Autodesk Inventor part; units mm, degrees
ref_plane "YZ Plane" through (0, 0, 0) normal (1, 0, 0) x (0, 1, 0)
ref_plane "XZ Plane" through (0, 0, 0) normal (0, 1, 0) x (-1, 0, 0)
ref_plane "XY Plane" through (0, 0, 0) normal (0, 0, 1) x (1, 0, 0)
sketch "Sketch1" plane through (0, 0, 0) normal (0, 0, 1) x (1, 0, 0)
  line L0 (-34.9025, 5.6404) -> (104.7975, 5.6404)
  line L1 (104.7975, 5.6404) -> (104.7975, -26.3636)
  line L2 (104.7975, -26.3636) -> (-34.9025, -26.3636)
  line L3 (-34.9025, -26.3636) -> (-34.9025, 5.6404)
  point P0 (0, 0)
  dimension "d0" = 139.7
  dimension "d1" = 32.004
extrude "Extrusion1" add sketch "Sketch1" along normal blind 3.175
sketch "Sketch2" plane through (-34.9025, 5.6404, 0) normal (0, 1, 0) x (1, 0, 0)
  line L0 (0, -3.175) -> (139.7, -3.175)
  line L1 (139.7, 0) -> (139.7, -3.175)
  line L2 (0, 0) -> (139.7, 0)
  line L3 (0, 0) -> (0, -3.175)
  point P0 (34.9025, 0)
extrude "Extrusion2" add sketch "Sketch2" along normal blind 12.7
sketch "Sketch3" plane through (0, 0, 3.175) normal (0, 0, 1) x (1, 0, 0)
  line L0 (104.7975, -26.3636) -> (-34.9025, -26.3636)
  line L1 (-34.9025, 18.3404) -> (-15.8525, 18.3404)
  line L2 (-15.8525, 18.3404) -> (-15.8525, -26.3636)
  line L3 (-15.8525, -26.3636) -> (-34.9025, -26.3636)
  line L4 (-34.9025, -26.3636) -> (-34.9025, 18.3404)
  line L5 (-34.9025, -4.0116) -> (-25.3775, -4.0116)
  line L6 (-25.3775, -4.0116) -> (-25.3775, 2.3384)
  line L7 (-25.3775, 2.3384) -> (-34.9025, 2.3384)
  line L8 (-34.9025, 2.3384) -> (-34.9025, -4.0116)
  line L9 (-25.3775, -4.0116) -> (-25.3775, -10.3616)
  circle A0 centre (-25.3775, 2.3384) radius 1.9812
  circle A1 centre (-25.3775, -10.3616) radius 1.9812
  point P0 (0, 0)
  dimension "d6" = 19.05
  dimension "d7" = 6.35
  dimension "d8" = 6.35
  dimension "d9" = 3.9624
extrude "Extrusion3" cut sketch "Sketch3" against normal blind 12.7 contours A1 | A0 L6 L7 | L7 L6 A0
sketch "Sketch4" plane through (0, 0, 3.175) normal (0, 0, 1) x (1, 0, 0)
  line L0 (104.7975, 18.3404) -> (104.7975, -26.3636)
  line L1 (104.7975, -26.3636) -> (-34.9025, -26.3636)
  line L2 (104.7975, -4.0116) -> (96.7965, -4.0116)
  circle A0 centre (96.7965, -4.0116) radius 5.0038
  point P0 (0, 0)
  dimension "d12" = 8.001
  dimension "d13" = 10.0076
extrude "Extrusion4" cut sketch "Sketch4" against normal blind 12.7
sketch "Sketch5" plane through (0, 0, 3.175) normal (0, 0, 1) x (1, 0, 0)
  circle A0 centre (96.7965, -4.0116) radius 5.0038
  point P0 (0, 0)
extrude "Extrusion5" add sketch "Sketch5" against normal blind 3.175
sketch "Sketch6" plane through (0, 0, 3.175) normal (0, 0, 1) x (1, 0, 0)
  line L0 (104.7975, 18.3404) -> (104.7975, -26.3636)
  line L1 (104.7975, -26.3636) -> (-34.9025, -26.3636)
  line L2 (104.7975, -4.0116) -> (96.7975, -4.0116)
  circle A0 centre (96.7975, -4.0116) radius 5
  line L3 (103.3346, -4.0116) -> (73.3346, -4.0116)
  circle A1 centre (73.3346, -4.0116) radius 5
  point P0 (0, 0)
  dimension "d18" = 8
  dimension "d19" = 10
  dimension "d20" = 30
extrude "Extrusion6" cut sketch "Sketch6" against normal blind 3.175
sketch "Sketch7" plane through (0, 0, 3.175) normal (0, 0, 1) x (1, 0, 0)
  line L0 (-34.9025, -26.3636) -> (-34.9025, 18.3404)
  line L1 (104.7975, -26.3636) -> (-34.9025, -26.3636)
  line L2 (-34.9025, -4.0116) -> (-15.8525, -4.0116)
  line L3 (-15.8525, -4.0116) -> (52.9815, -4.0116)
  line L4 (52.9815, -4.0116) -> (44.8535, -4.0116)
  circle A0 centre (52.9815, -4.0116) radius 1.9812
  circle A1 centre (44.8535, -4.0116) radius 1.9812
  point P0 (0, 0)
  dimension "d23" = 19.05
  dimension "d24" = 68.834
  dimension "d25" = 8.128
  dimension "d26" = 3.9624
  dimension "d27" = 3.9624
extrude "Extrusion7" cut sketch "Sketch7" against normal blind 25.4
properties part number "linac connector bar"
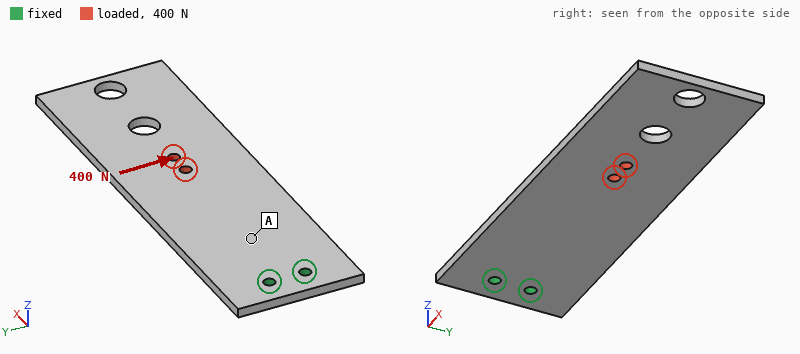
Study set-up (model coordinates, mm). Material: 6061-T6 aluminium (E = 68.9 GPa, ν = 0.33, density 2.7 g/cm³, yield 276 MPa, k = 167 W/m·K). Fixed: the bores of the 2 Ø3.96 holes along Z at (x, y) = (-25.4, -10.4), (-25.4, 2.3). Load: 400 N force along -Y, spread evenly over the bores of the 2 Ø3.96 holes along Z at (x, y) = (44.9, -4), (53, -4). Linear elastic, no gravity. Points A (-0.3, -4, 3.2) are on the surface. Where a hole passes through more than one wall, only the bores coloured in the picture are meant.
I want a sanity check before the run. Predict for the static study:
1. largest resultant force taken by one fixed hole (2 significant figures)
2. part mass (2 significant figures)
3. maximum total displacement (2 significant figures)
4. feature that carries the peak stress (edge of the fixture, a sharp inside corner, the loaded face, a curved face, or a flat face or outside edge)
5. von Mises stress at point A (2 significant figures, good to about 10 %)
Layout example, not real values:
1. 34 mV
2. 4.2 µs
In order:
1. 1.9 kN
2. 52 g
3. 0.18 mm
4. edge of the fixture
5. 9.0 MPa
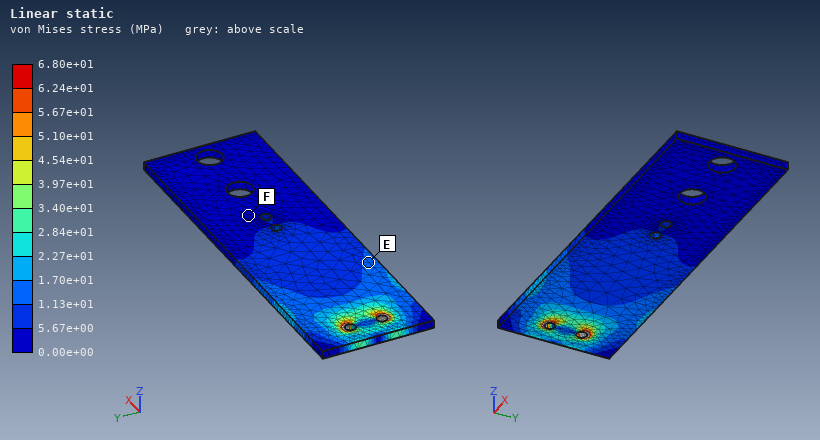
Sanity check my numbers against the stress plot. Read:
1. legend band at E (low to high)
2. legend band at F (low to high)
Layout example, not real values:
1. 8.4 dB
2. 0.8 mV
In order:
1. 1.13e+01 to 1.70e+01 MPa
2. 0.00e+00 to 5.67e+00 MPa
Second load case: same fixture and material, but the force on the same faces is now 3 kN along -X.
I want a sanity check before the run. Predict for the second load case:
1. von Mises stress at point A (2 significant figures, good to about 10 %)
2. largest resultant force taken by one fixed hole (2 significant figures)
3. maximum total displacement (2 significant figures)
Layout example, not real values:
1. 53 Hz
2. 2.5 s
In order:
1. 26 MPa
2. 1.5 kN
3. 33 µm
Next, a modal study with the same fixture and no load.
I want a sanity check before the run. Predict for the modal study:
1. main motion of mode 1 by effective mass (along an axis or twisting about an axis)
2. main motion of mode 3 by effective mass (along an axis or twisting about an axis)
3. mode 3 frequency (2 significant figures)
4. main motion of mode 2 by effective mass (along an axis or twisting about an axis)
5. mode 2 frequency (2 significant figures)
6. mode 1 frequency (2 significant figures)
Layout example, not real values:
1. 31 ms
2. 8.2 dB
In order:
1. along Z
2. along Z
3. 960 Hz
4. twisting about X
5. 860 Hz
6. 160 Hz
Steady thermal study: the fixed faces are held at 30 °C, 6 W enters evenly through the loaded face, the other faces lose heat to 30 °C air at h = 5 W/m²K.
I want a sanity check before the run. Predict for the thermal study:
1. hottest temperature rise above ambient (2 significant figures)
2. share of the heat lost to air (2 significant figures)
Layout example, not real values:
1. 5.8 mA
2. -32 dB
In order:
1. 19 K
2. 13 %
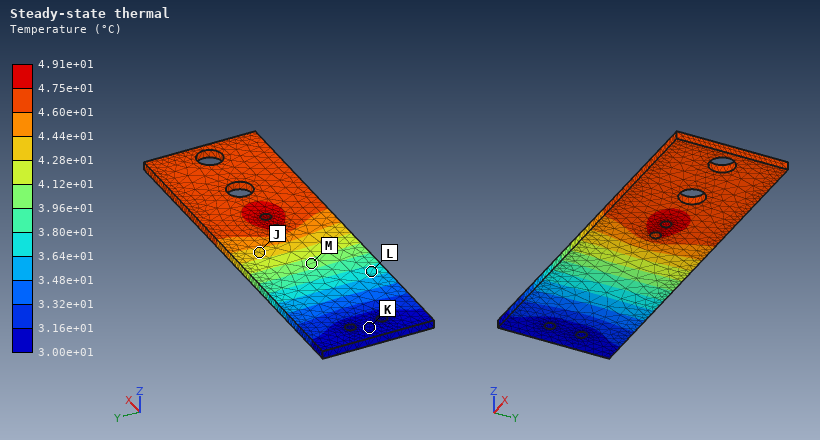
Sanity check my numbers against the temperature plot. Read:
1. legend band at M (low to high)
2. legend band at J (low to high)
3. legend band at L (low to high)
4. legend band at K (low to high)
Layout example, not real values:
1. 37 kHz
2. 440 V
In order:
1. 3.96e+01 to 4.12e+01 °C
2. 4.28e+01 to 4.44e+01 °C
3. 3.64e+01 to 3.80e+01 °C
4. 3.00e+01 to 3.16e+01 °C
